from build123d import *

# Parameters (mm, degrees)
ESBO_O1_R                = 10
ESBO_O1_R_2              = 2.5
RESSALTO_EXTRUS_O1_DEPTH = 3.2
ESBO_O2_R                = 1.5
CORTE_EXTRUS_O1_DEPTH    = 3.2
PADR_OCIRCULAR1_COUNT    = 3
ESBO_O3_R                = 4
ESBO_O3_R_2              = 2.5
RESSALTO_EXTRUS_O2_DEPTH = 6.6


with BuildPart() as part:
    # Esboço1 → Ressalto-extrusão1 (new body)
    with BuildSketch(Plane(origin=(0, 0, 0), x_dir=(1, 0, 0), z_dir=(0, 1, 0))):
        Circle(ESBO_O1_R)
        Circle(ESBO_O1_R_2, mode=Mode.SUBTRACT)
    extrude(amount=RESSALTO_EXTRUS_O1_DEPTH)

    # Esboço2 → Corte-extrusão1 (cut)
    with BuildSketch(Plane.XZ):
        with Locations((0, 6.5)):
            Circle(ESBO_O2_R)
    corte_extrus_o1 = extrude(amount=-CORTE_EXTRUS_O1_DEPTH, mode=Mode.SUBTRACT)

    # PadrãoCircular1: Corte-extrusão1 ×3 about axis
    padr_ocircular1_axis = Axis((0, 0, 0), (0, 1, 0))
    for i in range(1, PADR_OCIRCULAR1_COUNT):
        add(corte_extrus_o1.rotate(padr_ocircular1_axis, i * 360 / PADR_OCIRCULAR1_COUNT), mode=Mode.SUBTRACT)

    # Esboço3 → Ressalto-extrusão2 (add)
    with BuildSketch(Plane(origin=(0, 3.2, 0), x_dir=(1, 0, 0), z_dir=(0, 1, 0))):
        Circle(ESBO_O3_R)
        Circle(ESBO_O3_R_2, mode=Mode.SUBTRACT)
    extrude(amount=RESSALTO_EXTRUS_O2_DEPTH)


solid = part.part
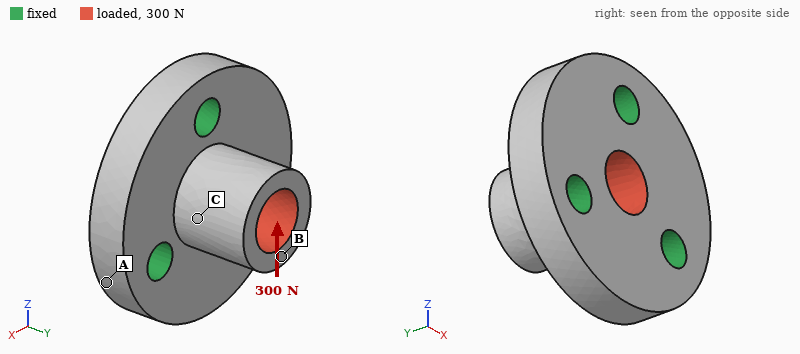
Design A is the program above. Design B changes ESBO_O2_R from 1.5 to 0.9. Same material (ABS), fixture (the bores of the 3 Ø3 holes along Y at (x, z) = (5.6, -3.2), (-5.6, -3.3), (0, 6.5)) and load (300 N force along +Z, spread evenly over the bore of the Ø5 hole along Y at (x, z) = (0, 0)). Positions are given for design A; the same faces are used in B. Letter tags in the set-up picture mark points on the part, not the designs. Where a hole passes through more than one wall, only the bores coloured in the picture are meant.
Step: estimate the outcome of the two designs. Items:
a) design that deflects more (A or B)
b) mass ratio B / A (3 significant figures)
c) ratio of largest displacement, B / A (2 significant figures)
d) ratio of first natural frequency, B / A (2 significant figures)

B
1.04
1.1
0.85
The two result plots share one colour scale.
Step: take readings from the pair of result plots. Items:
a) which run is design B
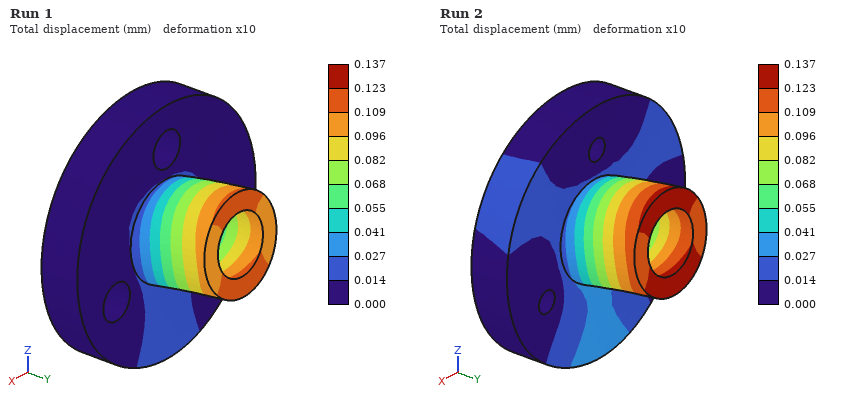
Run 2
